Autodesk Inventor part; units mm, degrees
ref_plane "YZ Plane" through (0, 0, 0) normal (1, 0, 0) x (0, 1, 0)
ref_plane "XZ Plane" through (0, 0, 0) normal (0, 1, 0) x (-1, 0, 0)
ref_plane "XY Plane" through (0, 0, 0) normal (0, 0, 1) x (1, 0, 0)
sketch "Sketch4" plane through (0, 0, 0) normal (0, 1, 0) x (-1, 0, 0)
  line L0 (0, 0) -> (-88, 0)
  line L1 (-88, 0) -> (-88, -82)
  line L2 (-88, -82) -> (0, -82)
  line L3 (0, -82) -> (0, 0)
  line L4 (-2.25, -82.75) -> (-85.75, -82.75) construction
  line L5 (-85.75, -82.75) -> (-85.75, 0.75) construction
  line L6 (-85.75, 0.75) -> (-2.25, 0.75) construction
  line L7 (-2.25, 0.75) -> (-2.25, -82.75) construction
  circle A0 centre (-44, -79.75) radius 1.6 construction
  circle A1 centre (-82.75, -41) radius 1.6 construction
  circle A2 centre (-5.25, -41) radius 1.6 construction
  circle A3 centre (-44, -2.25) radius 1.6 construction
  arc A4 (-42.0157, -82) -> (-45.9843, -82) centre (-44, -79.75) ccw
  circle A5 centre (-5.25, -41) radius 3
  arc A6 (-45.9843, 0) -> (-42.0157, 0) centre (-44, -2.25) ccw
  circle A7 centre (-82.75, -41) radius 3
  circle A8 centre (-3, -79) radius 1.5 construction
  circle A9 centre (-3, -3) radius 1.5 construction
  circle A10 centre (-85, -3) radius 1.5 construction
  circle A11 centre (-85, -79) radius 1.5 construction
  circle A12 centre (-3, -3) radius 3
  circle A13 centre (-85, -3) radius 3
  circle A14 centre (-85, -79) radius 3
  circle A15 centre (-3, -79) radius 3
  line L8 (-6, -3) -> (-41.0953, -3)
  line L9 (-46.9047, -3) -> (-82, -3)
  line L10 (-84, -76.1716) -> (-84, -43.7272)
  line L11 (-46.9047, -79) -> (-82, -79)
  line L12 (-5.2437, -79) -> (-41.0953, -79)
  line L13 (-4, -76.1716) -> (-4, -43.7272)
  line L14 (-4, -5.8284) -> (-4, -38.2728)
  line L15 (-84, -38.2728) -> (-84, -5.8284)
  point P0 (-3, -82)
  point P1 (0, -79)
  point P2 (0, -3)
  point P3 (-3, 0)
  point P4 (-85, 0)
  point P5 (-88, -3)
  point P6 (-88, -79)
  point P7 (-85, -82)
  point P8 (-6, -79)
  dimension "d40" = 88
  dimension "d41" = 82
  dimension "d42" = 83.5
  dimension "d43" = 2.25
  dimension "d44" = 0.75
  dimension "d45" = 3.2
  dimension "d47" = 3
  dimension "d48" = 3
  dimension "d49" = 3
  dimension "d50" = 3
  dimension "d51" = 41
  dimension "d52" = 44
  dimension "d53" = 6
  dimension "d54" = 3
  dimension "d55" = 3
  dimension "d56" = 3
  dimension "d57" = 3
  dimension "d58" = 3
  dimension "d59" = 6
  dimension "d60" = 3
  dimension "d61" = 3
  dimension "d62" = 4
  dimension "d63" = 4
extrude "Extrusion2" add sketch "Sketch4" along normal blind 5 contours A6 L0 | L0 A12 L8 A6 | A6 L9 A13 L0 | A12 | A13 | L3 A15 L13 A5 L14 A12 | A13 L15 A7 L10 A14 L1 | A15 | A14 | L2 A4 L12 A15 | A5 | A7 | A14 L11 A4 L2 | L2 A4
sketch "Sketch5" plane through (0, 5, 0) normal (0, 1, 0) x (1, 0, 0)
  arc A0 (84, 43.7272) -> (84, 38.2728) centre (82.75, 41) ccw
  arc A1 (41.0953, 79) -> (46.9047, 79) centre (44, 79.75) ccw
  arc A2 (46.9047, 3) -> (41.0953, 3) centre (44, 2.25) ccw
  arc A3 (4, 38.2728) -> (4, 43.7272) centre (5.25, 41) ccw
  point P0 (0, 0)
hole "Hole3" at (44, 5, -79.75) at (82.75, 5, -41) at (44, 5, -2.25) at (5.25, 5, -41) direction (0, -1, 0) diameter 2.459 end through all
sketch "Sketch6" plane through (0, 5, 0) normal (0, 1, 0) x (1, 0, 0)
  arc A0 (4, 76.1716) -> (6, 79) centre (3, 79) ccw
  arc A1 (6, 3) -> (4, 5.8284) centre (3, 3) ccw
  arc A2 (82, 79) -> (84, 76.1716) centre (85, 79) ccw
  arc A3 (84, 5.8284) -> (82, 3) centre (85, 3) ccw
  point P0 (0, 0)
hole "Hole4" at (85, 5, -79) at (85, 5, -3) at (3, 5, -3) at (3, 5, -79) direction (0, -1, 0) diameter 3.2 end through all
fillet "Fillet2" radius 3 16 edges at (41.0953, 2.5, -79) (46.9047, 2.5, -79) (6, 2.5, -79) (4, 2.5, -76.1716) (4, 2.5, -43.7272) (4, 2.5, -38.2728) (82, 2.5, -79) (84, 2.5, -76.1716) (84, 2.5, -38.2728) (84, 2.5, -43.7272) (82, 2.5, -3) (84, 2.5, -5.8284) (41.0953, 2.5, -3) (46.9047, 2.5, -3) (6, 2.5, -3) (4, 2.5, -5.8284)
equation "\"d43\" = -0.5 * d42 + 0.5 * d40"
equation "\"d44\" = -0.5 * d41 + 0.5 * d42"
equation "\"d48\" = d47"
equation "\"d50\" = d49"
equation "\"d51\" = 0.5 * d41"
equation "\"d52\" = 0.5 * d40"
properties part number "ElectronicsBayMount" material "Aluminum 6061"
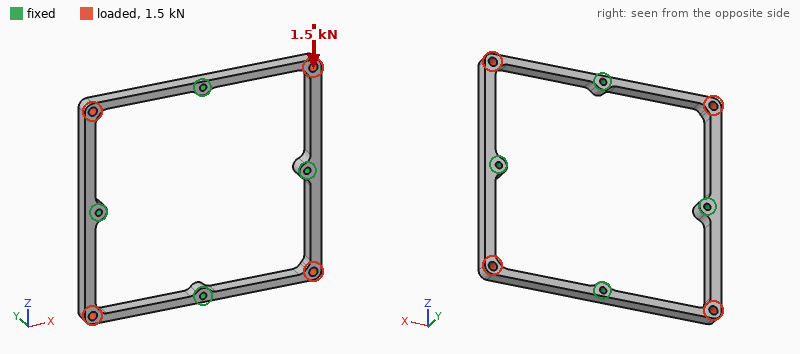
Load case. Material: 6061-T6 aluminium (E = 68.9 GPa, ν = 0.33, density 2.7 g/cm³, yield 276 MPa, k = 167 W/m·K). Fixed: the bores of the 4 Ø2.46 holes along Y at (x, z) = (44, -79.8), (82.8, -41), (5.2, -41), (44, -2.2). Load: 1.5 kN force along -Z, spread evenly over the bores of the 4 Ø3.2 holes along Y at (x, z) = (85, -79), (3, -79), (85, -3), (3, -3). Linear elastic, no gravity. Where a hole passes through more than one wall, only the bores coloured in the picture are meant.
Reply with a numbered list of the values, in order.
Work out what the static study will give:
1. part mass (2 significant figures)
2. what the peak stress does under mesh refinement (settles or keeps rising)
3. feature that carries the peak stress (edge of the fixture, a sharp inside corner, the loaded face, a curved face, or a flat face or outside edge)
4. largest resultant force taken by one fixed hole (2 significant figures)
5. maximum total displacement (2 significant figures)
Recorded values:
1. 16 g
2. keeps rising
3. edge of the fixture
4. 740 N
5. 22 µm
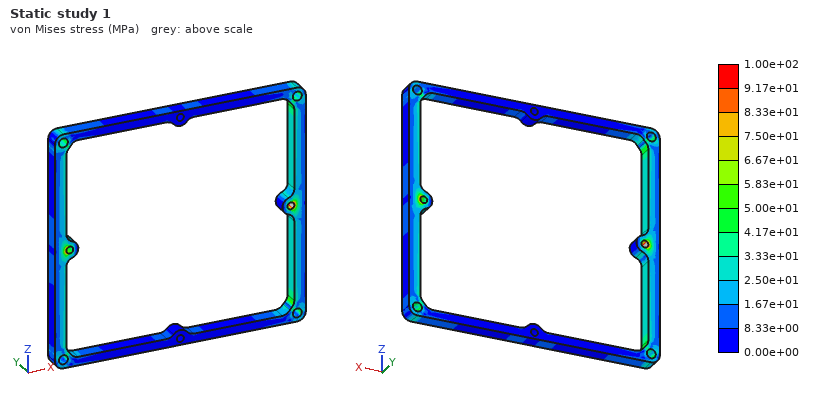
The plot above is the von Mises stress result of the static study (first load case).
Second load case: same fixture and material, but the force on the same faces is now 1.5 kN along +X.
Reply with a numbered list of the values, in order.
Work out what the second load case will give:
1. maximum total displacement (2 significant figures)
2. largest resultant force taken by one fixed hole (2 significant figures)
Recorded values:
1. 22 µm
2. 710 N
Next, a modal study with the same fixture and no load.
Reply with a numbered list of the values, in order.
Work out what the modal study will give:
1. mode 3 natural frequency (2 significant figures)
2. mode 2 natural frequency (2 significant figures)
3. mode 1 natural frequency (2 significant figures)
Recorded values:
1. 3000 Hz
2. 2900 Hz
3. 2900 Hz
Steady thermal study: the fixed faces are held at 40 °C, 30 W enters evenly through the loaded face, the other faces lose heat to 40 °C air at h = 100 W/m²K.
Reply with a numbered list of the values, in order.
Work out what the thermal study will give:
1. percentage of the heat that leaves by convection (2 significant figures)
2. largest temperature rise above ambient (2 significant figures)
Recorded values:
1. 32 %
2. 39 K
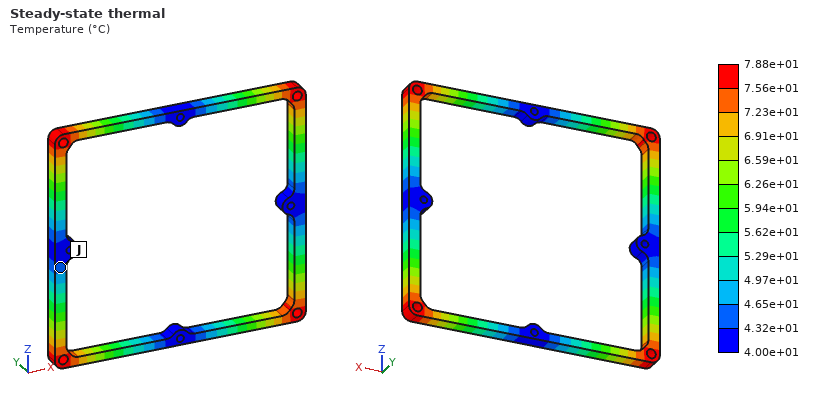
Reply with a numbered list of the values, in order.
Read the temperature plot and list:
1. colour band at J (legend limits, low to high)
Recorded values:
1. 4.32e+01 to 4.65e+01 °C
